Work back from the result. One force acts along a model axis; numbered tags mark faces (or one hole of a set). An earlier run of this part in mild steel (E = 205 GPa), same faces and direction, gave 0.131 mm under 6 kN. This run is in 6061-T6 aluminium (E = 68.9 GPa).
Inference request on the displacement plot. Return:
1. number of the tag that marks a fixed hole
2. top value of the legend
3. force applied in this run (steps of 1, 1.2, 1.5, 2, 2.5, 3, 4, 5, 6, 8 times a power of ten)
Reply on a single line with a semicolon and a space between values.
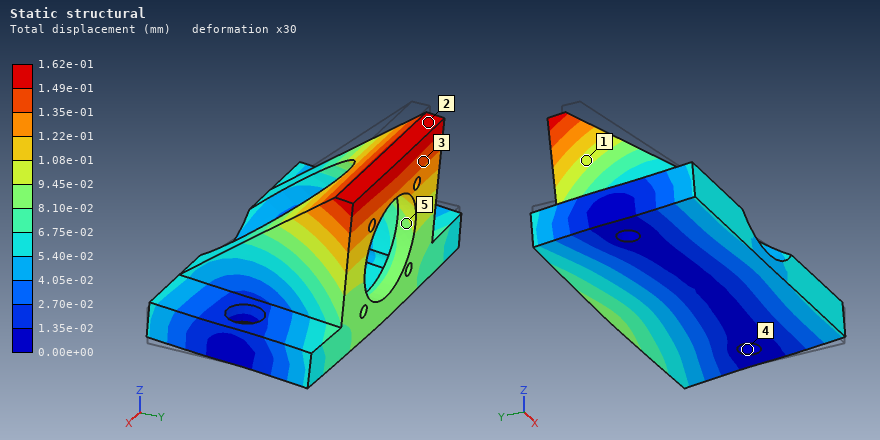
4; 1.62e-01 mm; 2.5 kN
